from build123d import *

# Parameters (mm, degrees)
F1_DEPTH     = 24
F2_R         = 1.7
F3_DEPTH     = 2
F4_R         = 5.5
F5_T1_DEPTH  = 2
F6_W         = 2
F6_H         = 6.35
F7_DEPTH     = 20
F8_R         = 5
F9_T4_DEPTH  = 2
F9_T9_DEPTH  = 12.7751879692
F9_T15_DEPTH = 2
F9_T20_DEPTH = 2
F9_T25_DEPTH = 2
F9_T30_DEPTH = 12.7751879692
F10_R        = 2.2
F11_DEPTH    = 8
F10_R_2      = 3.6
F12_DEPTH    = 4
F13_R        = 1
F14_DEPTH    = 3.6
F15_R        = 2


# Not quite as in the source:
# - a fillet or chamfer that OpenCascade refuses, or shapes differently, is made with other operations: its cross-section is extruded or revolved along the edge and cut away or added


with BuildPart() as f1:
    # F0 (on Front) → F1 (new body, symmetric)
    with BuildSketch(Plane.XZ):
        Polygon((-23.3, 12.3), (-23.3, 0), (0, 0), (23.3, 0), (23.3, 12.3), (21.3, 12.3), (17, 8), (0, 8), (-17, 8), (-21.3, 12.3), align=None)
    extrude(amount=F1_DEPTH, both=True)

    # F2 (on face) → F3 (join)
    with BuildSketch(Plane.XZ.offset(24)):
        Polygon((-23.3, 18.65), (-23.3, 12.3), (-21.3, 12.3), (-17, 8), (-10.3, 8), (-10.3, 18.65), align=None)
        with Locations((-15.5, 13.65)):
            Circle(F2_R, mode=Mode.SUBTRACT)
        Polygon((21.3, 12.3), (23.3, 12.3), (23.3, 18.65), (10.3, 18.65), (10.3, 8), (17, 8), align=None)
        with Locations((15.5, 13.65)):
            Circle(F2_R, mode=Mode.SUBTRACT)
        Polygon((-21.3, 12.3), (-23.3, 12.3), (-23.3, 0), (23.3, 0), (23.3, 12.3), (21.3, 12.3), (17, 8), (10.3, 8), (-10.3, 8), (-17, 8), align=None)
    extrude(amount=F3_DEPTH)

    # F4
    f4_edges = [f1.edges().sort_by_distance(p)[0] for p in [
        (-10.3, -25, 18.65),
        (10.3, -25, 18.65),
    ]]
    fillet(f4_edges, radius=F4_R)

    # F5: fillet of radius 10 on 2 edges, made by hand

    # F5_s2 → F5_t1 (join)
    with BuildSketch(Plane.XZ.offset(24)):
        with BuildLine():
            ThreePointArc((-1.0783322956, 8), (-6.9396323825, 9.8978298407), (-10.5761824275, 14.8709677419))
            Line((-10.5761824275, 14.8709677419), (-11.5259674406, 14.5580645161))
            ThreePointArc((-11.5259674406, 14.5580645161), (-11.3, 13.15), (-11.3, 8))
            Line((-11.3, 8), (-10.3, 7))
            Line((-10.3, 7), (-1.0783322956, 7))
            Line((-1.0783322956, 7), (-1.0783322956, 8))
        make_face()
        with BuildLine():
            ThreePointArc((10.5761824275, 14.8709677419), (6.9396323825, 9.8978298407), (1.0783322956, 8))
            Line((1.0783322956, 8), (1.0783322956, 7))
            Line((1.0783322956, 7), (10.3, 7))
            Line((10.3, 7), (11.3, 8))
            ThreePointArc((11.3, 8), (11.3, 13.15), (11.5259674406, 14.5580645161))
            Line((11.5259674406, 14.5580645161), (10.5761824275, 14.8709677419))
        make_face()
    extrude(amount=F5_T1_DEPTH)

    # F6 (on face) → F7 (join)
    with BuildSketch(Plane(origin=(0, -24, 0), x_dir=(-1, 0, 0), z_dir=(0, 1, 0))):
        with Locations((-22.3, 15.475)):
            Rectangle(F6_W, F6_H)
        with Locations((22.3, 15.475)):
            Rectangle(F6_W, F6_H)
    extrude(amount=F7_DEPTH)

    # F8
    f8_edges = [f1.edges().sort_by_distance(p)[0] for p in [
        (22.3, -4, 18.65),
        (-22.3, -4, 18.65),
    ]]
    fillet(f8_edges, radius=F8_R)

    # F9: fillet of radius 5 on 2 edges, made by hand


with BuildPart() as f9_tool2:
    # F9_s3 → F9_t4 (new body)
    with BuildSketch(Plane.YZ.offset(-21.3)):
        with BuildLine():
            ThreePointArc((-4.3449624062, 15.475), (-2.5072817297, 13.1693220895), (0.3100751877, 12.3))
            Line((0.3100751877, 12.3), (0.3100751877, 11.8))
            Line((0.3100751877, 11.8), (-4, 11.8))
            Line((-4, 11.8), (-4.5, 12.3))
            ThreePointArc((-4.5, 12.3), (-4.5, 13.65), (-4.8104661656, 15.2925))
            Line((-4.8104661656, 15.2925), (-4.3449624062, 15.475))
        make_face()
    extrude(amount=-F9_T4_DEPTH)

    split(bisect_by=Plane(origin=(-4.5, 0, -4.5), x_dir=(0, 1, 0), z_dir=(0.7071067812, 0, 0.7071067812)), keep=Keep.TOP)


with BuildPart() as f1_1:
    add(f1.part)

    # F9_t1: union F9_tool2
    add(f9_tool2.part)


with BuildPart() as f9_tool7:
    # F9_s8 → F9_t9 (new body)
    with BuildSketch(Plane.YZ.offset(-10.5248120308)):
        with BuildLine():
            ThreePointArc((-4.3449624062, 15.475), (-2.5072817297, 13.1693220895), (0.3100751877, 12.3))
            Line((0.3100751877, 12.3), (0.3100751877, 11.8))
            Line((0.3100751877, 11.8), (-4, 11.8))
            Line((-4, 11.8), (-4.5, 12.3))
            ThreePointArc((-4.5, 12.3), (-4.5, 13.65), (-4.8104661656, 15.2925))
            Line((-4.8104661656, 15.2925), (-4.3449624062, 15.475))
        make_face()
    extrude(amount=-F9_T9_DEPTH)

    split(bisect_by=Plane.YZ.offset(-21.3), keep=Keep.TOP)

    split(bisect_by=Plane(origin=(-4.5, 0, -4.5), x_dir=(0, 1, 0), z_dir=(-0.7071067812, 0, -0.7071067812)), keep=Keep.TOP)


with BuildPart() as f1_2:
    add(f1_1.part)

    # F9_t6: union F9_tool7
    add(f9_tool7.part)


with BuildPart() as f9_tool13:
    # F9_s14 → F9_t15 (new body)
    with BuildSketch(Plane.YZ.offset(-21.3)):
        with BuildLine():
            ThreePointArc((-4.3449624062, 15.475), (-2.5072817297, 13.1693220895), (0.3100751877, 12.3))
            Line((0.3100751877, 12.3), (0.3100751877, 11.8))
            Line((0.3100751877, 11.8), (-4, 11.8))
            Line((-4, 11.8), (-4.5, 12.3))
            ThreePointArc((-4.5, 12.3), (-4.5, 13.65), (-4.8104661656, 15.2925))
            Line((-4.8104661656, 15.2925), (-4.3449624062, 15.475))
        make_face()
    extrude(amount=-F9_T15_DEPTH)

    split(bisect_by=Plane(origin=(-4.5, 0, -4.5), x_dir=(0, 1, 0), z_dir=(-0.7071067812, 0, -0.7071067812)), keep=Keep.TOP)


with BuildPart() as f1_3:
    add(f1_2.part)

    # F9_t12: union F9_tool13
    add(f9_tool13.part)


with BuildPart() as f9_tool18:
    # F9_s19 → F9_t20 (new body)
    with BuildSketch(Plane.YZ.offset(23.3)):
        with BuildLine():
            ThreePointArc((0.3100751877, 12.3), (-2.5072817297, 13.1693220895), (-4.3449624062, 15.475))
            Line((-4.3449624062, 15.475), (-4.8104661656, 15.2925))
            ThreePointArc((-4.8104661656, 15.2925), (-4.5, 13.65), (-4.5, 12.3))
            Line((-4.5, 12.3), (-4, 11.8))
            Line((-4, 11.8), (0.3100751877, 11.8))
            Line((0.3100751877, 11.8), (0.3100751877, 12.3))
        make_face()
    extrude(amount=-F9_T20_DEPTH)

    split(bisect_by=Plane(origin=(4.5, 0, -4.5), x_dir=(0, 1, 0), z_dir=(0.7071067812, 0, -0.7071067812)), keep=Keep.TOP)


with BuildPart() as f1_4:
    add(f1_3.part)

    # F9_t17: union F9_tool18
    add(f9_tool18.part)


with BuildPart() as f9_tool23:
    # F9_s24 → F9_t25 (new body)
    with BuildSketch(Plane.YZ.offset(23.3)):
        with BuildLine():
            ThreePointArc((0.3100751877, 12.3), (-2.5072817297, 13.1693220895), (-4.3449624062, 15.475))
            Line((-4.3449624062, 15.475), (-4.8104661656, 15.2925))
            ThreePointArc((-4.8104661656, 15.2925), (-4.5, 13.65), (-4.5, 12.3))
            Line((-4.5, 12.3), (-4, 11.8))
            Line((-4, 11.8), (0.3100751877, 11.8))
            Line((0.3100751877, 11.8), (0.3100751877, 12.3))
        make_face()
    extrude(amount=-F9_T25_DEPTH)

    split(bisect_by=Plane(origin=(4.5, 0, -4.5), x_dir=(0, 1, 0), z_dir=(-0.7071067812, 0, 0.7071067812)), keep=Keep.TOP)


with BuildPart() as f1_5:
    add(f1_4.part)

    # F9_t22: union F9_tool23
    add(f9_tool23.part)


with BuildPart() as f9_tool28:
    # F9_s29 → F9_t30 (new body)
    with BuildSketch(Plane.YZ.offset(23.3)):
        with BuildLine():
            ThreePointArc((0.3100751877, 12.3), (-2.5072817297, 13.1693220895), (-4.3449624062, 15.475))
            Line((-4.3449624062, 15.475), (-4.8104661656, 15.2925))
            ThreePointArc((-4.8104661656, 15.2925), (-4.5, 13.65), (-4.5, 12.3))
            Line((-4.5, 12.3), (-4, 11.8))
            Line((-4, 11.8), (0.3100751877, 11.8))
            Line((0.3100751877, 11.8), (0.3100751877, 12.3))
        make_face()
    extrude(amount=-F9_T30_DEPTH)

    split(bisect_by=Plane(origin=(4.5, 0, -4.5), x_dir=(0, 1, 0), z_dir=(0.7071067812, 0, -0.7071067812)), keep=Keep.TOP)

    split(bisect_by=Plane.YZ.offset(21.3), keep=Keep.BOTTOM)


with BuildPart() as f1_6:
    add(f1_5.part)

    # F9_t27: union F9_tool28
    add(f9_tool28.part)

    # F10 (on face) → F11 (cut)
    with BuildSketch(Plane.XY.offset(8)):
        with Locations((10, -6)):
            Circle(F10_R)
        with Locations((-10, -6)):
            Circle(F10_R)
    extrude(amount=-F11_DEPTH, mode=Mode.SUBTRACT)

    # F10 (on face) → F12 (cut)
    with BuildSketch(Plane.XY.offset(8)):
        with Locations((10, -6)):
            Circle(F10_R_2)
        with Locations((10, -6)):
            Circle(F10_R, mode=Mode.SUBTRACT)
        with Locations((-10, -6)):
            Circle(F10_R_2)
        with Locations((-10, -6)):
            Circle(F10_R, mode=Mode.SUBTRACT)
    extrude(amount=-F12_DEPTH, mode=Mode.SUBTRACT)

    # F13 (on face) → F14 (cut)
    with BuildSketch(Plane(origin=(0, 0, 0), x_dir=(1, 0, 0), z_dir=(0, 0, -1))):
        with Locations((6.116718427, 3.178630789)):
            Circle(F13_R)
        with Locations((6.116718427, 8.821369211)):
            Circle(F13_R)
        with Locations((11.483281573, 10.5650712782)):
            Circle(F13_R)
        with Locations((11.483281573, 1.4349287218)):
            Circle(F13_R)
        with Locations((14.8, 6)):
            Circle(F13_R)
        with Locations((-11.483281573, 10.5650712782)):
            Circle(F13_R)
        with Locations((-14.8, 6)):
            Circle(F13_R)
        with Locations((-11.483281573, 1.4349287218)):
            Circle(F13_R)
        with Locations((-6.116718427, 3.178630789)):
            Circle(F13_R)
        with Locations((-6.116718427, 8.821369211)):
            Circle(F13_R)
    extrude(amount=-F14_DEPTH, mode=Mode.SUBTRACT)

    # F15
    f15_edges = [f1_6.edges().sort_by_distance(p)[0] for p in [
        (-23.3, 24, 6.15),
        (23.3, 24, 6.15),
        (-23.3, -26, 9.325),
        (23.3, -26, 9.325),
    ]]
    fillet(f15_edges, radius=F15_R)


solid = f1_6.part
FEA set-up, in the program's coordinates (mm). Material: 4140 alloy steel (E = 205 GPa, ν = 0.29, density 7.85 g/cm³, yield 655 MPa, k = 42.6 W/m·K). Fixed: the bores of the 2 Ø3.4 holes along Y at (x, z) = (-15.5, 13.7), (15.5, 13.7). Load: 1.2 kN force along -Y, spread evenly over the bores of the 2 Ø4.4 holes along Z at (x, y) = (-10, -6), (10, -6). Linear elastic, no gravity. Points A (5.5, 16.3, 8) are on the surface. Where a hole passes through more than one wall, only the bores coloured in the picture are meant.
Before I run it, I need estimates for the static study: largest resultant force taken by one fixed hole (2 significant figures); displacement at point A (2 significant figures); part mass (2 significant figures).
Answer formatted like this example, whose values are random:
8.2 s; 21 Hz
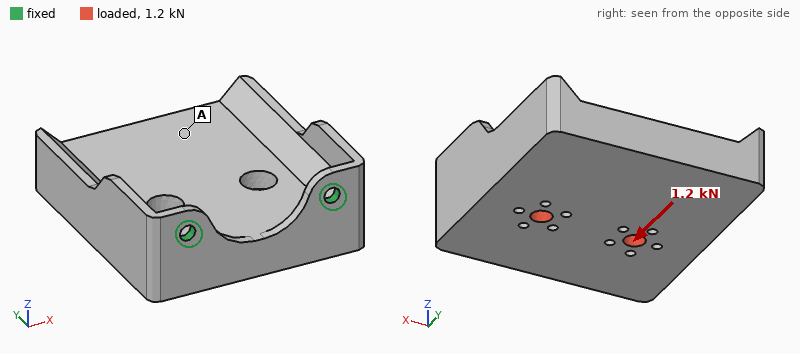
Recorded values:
610 N; 0.26 mm; 160 g
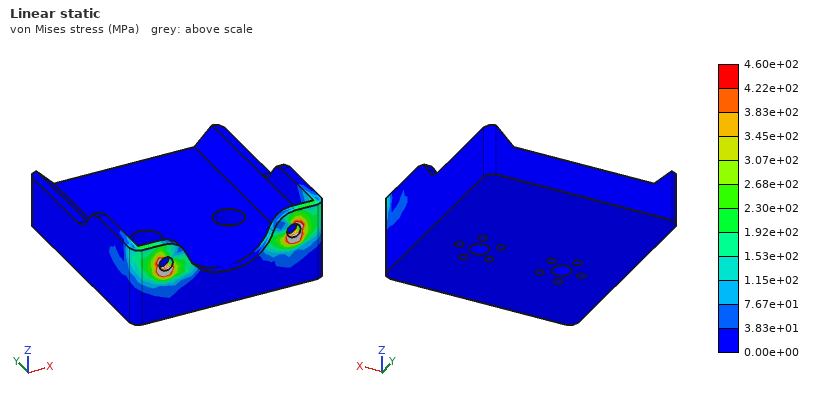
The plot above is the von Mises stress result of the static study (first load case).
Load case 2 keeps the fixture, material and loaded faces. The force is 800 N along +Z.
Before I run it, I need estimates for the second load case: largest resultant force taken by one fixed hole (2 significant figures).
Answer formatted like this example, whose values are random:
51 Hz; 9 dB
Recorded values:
410 N
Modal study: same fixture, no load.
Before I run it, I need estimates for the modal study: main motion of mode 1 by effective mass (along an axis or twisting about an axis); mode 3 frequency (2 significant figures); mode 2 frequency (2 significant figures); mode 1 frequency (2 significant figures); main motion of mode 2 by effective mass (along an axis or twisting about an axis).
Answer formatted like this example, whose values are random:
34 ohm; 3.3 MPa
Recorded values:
along Z; 5000 Hz; 2600 Hz; 580 Hz; along X
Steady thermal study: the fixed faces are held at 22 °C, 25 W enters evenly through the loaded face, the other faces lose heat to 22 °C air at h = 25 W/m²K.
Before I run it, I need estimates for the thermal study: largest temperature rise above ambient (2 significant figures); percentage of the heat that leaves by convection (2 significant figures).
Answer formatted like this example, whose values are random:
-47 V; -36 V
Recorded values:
70 K; 38 %
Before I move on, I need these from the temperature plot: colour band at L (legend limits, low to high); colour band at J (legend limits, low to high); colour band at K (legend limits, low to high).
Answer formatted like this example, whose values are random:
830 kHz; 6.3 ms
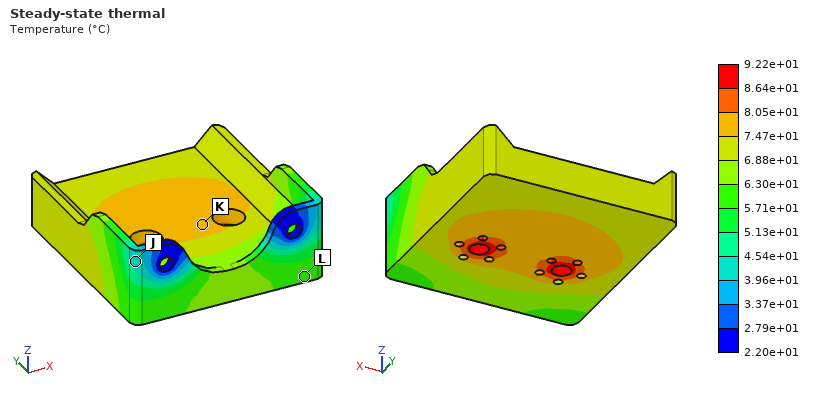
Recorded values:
5.71e+01 to 6.30e+01 °C; 3.96e+01 to 4.54e+01 °C; 7.47e+01 to 8.05e+01 °C
